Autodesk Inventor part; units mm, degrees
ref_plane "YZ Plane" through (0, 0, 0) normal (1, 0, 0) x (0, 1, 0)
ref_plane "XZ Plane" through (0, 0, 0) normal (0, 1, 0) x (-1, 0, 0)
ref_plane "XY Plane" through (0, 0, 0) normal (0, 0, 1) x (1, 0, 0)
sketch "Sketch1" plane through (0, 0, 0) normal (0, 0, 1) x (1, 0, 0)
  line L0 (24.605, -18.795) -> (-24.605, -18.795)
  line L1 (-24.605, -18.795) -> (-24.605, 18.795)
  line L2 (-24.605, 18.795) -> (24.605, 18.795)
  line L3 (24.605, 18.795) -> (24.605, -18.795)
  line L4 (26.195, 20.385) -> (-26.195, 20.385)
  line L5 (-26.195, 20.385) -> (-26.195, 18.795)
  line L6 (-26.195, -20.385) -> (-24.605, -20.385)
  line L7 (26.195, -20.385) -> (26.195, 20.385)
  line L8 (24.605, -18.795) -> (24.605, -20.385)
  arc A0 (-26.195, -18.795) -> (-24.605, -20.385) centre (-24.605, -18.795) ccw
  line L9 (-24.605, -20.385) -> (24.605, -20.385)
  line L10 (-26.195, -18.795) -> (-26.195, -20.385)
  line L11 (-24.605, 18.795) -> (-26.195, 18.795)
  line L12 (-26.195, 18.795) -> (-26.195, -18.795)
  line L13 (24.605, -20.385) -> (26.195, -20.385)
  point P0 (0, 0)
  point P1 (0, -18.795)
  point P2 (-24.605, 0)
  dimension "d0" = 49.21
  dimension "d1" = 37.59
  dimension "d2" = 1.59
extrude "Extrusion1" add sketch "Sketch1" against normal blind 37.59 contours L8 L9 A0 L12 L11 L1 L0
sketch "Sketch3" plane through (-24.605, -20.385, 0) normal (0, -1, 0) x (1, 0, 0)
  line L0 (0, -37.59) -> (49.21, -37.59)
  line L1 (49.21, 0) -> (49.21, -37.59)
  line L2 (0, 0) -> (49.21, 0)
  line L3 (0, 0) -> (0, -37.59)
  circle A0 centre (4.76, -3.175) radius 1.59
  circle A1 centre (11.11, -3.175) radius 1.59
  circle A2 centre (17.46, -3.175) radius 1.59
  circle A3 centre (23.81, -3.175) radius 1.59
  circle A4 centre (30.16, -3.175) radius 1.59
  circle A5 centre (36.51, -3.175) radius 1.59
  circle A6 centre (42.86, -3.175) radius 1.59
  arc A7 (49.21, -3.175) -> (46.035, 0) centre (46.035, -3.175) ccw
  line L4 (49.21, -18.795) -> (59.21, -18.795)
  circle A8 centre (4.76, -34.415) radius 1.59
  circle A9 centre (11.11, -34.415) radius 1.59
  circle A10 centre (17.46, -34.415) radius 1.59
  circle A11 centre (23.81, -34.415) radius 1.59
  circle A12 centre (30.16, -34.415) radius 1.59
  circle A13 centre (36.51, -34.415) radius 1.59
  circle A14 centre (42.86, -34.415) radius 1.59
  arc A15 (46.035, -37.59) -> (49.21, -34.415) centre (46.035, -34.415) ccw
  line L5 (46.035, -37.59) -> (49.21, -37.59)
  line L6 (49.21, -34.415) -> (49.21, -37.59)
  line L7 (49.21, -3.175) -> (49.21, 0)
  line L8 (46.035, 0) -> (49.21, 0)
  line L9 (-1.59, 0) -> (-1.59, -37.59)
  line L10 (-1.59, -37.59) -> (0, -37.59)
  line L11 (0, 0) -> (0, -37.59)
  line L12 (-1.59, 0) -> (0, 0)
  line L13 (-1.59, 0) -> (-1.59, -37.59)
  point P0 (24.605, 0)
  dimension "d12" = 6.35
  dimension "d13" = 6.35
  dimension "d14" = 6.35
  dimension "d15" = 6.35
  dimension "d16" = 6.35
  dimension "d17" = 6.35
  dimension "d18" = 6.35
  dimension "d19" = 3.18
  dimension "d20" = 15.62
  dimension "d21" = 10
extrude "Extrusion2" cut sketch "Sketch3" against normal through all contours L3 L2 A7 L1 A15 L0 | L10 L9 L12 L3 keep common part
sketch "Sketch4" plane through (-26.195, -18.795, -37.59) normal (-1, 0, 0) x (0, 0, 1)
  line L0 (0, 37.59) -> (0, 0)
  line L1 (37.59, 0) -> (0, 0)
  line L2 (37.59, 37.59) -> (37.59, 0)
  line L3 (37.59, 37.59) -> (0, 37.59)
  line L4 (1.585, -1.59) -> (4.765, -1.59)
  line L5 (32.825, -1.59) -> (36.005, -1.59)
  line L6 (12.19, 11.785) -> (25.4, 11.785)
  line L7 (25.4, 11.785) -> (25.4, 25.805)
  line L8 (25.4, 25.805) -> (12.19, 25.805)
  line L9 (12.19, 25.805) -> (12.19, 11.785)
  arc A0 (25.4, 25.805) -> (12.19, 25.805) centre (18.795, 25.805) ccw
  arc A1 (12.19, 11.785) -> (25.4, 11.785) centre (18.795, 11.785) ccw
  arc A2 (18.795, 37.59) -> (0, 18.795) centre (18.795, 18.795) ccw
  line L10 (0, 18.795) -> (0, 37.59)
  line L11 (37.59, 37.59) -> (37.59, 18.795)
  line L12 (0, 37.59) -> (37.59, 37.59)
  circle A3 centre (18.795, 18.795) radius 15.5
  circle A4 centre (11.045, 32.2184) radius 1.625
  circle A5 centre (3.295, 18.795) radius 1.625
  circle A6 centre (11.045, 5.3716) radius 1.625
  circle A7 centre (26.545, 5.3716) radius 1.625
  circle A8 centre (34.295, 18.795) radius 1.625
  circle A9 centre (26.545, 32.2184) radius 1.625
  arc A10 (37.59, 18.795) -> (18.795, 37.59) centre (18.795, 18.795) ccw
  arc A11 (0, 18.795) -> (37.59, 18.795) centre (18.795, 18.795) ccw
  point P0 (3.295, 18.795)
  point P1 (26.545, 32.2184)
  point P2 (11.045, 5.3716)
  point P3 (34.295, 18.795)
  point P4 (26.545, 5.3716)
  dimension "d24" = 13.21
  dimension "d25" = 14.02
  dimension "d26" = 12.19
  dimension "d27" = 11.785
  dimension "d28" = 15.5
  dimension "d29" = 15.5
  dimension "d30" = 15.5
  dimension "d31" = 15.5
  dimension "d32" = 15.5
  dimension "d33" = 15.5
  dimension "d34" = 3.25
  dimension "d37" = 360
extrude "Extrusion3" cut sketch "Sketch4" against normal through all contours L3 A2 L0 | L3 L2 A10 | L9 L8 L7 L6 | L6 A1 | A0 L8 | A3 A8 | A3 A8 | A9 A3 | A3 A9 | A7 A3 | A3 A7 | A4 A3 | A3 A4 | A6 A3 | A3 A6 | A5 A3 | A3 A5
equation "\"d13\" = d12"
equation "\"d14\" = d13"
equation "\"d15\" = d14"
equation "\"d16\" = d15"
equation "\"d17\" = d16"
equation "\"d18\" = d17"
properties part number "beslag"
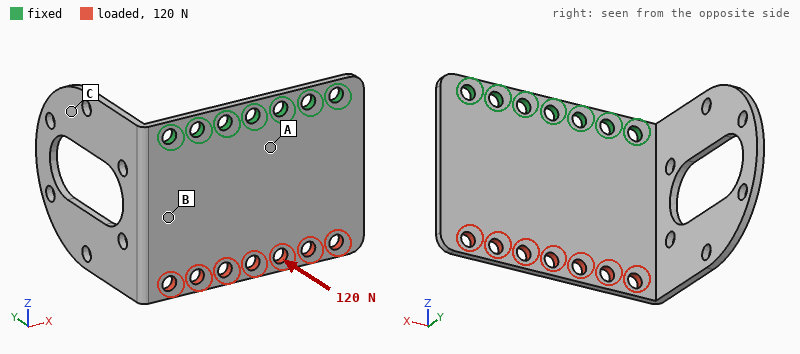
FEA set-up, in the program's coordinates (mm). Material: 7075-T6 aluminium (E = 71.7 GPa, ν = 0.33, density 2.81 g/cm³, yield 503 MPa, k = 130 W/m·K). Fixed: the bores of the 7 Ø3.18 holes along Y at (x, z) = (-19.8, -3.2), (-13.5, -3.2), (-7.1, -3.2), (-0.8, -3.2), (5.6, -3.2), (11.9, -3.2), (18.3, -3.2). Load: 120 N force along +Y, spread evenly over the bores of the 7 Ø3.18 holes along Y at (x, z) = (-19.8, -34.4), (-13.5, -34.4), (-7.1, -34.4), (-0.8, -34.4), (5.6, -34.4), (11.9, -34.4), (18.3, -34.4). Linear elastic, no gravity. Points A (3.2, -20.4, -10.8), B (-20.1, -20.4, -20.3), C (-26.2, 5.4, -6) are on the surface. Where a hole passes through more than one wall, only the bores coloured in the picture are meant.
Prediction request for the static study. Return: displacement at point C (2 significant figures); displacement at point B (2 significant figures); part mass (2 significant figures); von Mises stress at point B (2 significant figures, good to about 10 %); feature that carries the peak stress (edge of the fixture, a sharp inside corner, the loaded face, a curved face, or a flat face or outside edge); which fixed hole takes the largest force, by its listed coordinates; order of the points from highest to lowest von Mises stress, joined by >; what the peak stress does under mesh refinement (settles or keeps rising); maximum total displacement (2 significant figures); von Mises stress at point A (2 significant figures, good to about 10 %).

0.27 mm
0.18 mm
12 g
48 MPa
edge of the fixture
(-19.8, -3.2)
A > B > C
keeps rising
0.78 mm
92 MPa
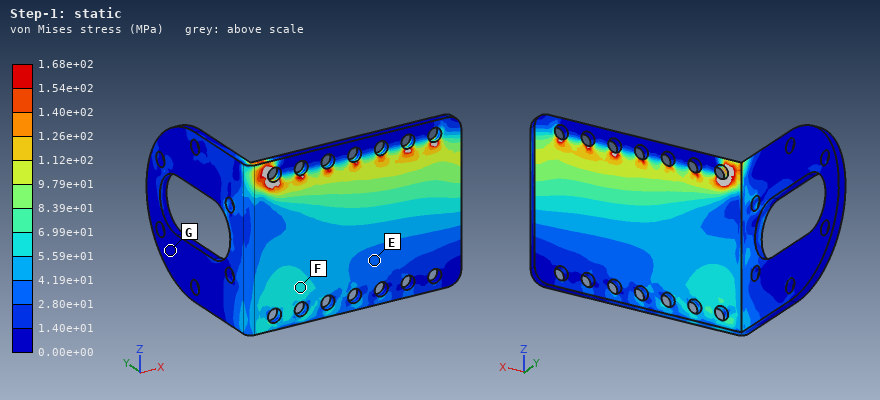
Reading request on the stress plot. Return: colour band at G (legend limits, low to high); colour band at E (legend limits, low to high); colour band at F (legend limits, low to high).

0.00e+00 to 1.40e+01 MPa
2.80e+01 to 4.19e+01 MPa
5.59e+01 to 6.99e+01 MPa
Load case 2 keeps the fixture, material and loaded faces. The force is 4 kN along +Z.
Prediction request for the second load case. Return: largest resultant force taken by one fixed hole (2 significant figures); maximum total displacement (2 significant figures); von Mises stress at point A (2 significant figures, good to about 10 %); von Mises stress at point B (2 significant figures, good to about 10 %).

780 N
27 µm
52 MPa
41 MPa
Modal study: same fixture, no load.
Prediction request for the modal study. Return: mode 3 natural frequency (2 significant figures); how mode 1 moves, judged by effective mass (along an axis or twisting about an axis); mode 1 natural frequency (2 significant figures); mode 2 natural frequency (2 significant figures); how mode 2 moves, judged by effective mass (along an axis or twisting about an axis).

1700 Hz
along X
770 Hz
1100 Hz
along Y
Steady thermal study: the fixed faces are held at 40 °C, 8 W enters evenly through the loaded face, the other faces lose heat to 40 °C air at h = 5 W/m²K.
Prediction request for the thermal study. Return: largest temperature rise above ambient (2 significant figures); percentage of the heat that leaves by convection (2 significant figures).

24 K
3.6 %
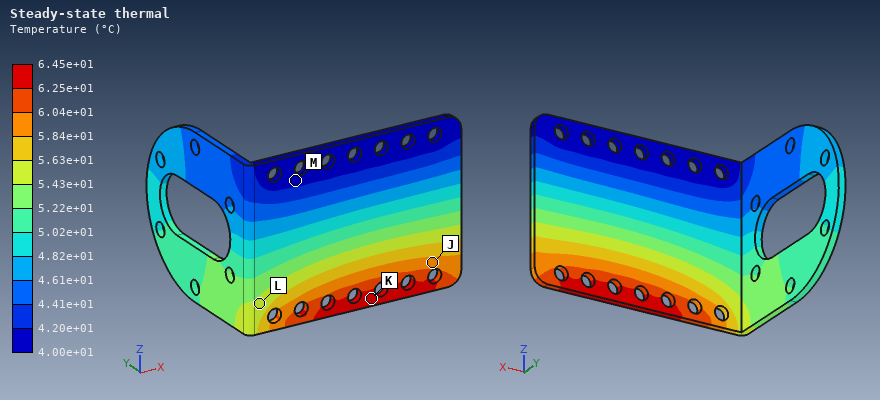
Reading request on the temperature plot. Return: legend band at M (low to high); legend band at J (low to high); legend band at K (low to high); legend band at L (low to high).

4.00e+01 to 4.20e+01 °C
5.84e+01 to 6.04e+01 °C
6.25e+01 to 6.45e+01 °C
5.43e+01 to 5.63e+01 °C
